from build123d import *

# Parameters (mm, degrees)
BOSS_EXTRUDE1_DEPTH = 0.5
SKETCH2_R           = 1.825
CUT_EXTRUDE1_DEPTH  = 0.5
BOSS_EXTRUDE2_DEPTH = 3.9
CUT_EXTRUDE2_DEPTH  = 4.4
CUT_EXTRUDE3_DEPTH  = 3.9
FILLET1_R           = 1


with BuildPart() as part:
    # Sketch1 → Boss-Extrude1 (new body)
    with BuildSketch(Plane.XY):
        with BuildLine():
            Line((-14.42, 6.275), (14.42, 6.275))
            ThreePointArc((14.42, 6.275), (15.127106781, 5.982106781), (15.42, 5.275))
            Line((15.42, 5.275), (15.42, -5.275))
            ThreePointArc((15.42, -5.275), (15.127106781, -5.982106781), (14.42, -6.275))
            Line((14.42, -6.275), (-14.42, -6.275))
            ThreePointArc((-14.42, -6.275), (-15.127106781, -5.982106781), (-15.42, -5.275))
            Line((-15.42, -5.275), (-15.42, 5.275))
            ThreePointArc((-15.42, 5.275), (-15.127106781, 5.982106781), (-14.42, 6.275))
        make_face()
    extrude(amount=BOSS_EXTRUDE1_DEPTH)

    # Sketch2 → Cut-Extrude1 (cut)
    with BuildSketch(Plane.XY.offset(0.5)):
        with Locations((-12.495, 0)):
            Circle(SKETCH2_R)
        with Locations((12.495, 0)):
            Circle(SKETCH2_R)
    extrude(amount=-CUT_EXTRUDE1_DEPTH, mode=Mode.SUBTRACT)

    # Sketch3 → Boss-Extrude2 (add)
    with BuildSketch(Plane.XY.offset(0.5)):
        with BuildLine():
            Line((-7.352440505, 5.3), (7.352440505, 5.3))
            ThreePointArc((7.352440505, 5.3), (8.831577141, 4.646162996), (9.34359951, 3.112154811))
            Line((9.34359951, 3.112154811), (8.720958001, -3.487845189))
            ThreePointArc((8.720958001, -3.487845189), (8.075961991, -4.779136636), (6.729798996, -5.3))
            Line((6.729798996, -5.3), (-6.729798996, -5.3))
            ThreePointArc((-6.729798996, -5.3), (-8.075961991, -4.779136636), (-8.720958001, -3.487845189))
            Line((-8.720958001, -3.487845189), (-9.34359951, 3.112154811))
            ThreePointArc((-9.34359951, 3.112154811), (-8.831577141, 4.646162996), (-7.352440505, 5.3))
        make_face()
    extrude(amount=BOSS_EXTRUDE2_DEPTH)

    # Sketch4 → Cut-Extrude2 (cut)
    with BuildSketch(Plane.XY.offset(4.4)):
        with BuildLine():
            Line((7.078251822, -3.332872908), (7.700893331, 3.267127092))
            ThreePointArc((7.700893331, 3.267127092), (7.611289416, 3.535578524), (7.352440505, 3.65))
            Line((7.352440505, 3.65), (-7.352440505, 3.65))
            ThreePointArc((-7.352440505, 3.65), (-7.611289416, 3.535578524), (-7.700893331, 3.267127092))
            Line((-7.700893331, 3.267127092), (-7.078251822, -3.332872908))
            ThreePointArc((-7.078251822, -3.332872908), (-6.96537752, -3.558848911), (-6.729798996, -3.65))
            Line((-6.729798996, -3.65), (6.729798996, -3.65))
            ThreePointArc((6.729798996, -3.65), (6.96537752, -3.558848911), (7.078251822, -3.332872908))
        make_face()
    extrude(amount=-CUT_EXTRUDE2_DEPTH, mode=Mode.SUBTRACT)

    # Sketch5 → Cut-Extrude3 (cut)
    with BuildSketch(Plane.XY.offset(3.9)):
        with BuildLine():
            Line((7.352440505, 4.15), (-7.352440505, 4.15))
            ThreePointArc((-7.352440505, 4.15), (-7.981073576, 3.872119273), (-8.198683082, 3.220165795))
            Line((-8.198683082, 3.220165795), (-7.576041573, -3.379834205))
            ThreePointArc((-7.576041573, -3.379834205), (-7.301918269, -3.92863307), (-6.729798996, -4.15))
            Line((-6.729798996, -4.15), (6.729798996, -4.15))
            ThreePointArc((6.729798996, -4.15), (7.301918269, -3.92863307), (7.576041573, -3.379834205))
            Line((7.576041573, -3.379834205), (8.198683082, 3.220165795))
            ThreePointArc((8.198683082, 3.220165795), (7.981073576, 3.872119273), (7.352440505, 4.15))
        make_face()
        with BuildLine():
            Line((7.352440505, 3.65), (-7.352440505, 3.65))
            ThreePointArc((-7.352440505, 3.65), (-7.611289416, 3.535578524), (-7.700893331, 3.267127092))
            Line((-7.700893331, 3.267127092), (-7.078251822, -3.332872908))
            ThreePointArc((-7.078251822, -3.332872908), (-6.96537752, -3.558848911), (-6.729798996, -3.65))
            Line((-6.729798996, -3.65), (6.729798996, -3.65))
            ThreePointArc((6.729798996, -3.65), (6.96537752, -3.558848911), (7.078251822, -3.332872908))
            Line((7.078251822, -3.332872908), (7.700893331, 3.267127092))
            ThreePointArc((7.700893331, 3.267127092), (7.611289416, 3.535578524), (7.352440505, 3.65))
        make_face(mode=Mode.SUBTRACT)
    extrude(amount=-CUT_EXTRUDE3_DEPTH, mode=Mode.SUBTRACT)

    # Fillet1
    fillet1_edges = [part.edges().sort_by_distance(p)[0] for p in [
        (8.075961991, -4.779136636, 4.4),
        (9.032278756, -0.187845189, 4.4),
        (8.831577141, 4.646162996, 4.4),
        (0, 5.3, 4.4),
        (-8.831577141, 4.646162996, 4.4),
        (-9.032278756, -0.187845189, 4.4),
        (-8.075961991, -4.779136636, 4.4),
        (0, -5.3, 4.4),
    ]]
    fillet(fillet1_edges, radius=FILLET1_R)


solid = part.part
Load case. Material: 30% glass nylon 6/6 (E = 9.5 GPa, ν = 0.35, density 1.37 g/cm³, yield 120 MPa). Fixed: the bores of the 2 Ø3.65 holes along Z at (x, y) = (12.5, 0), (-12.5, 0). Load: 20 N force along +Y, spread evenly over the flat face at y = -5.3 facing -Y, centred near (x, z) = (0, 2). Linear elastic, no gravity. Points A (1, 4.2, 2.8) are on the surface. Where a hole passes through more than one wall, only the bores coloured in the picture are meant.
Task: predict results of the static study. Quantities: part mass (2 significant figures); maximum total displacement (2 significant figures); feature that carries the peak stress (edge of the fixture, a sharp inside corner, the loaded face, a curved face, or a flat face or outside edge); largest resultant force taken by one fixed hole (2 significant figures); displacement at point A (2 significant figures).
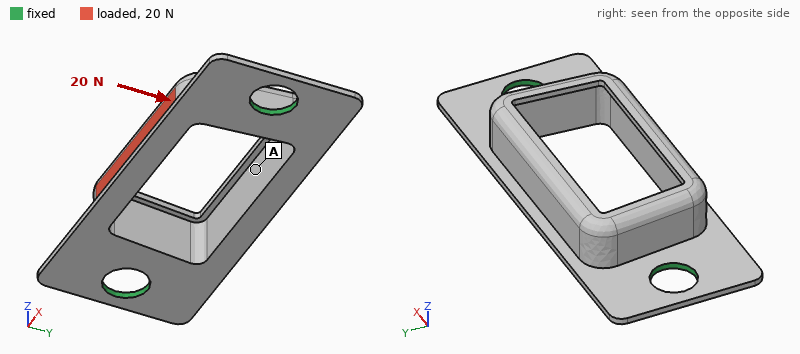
0.47 g
90 µm
a curved face
11 N
38 µm
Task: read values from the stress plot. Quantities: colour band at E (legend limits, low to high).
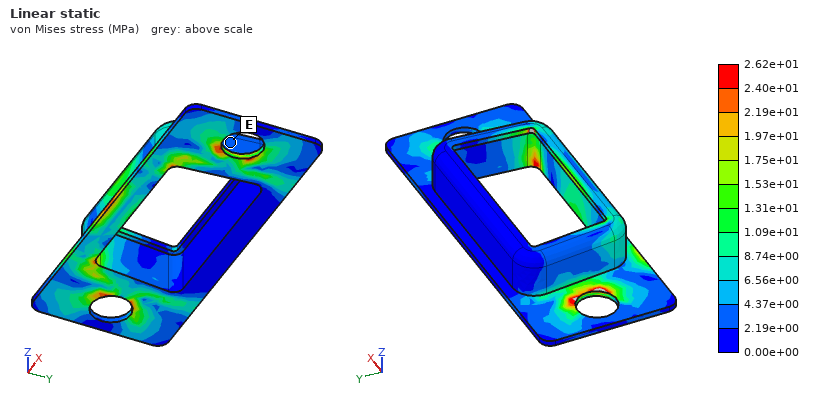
2.19e+00 to 4.37e+00 MPa
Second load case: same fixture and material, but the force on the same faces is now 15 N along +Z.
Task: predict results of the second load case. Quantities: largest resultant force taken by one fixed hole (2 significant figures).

11 N
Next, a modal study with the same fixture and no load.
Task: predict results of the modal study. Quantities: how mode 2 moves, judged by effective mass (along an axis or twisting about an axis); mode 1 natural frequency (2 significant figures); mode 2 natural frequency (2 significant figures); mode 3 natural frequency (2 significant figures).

along Z
3400 Hz
7800 Hz
8700 Hz
